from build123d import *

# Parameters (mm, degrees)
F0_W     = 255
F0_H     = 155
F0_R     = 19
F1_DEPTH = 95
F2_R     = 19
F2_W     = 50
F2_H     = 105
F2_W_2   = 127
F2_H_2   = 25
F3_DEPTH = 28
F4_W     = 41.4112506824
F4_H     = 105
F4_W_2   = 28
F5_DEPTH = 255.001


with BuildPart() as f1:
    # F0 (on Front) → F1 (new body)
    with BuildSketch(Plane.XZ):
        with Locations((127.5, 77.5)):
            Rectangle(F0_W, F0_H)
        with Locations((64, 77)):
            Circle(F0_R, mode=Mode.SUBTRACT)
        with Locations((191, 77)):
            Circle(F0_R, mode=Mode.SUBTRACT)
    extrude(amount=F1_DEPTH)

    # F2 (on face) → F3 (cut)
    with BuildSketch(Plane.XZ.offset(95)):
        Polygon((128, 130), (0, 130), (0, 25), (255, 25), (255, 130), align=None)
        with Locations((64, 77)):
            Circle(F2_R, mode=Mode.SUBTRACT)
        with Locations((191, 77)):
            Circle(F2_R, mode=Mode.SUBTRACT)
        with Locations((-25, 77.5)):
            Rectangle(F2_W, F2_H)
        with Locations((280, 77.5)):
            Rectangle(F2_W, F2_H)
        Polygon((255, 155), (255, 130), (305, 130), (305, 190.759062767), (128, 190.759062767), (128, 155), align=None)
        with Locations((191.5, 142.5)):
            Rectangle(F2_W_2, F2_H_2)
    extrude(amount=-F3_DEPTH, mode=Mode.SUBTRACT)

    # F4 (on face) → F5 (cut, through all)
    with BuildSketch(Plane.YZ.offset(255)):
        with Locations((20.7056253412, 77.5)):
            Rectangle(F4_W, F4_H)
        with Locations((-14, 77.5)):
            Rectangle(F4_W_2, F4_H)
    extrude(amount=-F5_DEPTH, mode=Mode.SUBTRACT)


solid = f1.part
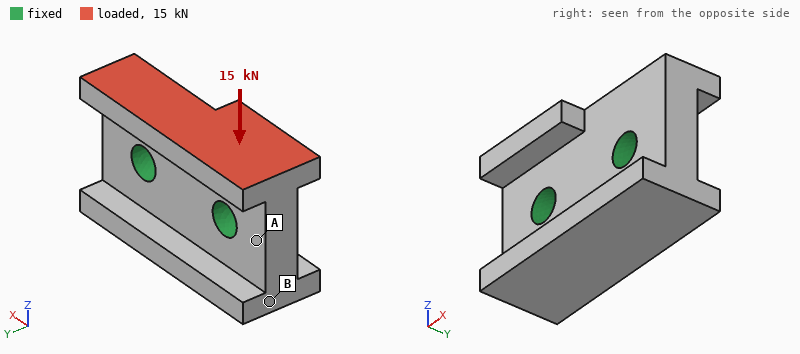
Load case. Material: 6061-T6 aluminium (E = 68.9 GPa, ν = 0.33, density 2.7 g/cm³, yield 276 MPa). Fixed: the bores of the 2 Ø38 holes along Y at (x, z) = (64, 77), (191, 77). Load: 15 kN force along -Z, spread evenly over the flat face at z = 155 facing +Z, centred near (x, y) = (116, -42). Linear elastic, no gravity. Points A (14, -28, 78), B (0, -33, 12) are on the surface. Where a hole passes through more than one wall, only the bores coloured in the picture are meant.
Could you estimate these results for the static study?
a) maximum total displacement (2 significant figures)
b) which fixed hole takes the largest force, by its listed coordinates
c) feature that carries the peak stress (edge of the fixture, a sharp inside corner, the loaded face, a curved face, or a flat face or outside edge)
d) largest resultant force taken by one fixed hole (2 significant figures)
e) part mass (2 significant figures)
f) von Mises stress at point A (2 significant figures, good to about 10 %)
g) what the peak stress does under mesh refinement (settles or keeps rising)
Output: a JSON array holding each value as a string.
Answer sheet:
["10 µm", "(64, 77)", "edge of the fixture", "8.7 kN", "5.6 kg", "0.99 MPa", "keeps rising"]
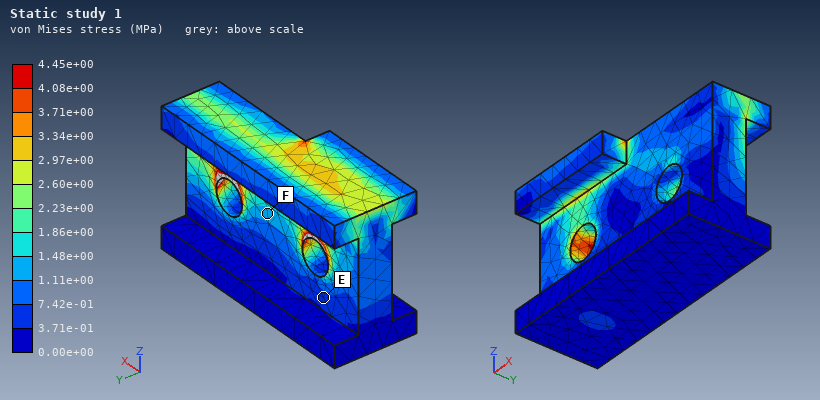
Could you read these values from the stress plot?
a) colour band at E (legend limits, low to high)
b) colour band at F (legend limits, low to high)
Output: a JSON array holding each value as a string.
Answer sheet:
["3.71e-01 to 7.42e-01 MPa", "1.11e+00 to 1.48e+00 MPa"]
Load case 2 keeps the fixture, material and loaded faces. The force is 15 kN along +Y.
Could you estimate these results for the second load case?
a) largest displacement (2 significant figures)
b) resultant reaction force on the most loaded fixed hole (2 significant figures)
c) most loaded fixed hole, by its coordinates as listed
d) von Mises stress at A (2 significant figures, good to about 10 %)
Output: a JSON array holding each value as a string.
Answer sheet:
["40 µm", "8.5 kN", "(64, 77)", "6.2 MPa"]
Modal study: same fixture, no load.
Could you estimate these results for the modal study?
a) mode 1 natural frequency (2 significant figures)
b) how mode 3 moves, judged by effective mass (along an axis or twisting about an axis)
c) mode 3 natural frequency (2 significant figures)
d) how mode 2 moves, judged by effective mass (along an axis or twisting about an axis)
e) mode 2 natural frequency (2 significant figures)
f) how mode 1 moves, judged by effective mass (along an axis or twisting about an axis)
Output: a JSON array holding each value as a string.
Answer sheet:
["3000 Hz", "along Y", "3600 Hz", "along Y", "3400 Hz", "twisting about X"]
